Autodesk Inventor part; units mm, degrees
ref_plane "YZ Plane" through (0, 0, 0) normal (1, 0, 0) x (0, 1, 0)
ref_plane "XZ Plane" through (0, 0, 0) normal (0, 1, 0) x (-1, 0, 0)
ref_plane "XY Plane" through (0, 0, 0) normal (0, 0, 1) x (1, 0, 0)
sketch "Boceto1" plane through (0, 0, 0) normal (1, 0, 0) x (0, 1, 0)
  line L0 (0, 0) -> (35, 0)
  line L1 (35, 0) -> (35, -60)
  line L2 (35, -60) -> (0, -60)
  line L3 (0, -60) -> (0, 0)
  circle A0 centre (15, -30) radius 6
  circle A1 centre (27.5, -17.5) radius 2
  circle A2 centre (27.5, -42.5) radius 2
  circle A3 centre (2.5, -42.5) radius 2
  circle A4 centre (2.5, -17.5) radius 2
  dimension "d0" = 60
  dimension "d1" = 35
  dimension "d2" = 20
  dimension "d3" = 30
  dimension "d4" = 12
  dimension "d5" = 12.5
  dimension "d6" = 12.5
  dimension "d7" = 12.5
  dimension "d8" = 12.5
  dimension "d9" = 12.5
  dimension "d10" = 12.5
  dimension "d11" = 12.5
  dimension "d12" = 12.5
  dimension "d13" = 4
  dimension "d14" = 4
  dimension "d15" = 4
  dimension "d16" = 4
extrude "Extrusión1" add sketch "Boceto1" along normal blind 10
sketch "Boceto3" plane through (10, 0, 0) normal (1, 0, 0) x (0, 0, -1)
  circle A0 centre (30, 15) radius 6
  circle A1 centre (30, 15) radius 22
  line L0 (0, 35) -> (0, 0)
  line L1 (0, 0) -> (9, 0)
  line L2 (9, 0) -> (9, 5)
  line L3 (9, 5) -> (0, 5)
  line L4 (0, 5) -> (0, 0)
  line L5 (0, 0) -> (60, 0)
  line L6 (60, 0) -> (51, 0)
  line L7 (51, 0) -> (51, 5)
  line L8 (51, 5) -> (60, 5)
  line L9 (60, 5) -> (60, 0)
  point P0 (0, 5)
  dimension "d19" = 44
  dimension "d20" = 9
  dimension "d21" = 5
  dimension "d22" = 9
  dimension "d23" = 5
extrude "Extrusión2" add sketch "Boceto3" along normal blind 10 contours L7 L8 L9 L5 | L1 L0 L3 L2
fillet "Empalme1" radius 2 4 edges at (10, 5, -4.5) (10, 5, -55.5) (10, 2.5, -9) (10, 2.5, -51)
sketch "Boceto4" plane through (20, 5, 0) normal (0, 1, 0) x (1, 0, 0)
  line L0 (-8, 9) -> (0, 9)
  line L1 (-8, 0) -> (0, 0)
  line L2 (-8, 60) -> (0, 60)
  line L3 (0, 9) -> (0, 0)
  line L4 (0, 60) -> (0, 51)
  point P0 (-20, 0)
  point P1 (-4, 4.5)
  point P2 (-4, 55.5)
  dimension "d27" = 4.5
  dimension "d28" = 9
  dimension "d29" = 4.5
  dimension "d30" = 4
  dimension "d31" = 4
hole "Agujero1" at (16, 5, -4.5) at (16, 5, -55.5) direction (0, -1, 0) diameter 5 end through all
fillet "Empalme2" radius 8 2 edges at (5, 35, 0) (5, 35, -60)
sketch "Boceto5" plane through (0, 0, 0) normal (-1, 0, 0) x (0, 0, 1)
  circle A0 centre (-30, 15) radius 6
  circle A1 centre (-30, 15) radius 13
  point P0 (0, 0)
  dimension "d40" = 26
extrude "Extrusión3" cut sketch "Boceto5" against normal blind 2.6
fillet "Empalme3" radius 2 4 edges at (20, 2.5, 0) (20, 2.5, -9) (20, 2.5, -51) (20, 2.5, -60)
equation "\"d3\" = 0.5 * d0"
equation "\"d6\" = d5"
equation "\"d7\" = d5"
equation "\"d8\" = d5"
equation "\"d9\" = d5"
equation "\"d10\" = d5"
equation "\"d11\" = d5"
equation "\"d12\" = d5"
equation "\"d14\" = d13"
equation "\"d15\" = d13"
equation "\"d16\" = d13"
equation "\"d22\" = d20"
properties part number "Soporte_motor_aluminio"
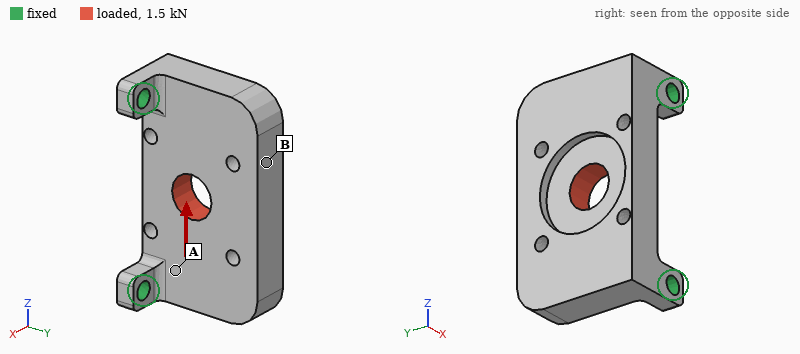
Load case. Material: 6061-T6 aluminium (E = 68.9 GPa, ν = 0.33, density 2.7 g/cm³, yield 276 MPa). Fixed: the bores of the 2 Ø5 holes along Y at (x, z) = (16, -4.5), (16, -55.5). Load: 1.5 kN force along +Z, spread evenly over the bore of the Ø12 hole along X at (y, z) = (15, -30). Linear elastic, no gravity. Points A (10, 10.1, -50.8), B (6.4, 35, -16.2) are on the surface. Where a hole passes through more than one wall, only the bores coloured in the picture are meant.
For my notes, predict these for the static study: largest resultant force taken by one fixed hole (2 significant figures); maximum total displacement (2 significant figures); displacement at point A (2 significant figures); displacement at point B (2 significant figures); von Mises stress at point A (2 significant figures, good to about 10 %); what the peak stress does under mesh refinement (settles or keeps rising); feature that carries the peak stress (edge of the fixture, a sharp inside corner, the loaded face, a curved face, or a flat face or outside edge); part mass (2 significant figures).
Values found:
840 N
17 µm
9.9 µm
16 µm
16 MPa
keeps rising
edge of the fixture
51 g
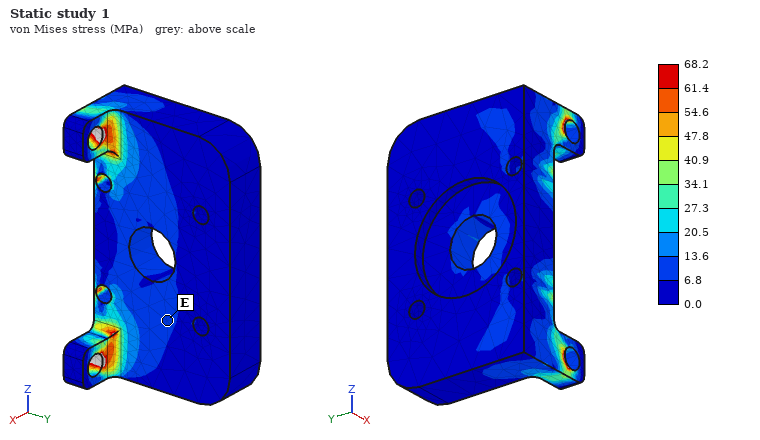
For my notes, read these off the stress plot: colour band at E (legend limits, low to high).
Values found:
6.8 to 13.6 MPa
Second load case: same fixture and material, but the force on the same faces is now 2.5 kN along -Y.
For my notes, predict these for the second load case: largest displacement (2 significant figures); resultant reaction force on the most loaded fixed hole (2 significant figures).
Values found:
0.20 mm
1.3 kN
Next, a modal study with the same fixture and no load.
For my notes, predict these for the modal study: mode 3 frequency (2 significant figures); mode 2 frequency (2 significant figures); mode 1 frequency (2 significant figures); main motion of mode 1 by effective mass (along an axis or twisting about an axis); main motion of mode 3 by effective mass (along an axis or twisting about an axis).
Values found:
8100 Hz
5900 Hz
1700 Hz
along X
along Z
